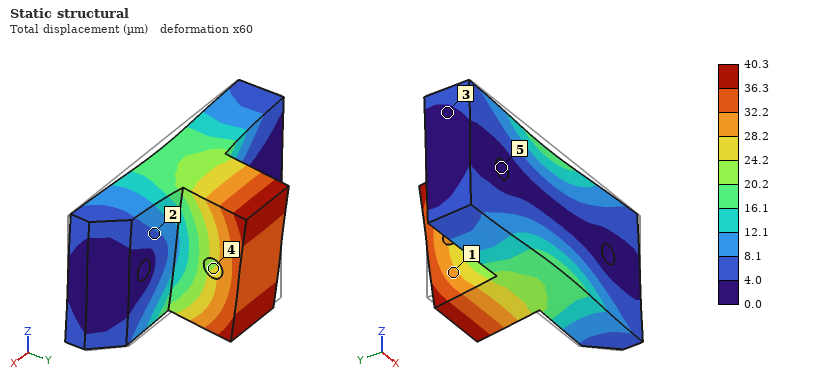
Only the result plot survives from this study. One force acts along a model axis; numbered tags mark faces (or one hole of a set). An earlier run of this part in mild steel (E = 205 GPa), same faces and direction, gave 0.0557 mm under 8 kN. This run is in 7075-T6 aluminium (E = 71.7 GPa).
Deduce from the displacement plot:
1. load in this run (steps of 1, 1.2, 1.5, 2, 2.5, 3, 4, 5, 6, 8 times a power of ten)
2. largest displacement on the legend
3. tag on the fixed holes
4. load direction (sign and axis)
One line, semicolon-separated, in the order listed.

2 kN; 40.3 µm; 5; -Z
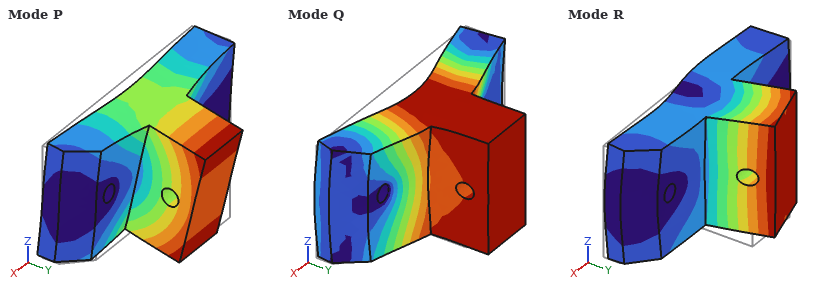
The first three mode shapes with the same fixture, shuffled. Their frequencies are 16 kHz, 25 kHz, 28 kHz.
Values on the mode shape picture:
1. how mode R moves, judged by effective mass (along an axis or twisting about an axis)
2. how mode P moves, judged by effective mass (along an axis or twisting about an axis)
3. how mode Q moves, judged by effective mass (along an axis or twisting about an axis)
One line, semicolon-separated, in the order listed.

along X; along Z; along Y
